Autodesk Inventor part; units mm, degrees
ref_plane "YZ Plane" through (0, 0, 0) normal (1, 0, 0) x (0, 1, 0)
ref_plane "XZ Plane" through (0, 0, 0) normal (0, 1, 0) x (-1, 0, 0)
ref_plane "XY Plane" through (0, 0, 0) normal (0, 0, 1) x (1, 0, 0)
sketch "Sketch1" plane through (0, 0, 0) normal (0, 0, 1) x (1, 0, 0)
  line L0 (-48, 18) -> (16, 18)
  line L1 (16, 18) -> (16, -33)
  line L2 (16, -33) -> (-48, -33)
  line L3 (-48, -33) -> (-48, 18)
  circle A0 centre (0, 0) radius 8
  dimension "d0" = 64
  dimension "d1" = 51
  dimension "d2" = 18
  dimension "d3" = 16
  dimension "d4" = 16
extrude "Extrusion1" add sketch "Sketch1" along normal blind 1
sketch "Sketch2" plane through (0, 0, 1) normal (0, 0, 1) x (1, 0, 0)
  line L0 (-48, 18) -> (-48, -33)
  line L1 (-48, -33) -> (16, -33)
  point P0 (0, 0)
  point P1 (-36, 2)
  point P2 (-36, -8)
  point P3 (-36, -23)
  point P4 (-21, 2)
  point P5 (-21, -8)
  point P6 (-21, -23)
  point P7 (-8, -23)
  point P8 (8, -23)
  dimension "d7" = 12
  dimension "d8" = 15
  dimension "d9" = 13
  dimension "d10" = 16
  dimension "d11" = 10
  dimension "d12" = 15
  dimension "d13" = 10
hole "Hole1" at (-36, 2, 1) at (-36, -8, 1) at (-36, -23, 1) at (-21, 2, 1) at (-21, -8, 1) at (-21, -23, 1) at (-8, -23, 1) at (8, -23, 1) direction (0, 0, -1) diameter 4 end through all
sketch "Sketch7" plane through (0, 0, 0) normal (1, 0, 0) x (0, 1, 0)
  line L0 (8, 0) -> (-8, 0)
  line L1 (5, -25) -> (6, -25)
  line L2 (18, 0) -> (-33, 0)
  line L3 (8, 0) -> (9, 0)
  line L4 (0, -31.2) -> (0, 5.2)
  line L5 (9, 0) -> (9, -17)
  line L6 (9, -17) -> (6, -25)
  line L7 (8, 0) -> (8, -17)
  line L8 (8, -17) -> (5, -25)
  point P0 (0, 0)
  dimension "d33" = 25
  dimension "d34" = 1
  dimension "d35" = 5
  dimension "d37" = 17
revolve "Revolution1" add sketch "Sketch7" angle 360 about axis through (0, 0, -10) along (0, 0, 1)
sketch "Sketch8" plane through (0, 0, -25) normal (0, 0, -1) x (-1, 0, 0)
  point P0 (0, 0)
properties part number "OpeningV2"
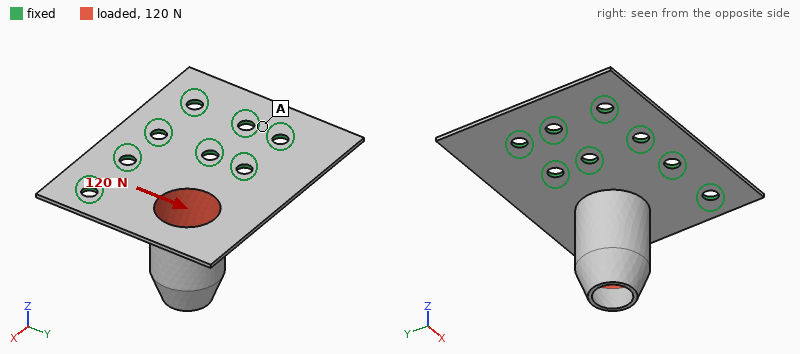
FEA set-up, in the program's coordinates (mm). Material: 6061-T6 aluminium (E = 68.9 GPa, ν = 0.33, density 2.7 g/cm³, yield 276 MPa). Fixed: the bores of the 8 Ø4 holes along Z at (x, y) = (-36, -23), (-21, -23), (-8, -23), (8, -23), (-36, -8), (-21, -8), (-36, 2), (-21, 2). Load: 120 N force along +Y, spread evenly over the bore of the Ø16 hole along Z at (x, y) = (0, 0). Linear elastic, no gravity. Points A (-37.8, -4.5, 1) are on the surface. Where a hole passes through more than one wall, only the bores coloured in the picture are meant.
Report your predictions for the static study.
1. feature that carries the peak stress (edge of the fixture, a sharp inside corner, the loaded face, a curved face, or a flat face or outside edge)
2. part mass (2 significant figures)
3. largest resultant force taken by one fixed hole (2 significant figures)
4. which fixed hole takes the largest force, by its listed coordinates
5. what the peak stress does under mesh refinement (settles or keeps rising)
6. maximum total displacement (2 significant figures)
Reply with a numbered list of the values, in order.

1. edge of the fixture
2. 11 g
3. 66 N
4. (8, -23)
5. keeps rising
6. 0.57 mm
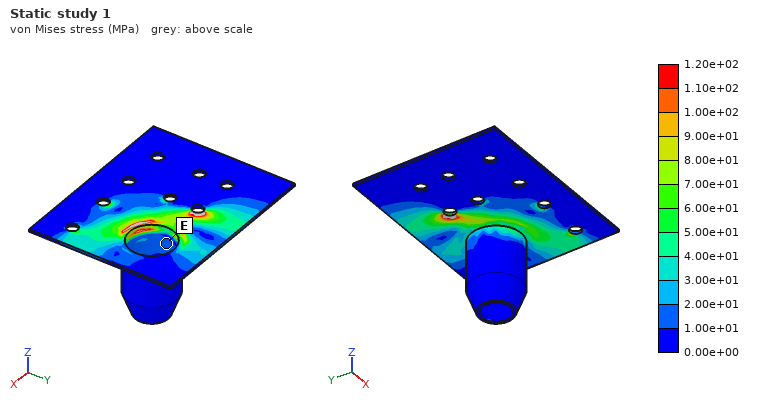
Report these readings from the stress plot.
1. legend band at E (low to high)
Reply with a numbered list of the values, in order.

1. 1.00e+01 to 2.00e+01 MPa
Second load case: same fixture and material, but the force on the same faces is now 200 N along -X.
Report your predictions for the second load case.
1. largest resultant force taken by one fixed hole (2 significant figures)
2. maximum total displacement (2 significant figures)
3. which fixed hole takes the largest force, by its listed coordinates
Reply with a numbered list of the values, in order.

1. 97 N
2. 0.92 mm
3. (-21, 2)
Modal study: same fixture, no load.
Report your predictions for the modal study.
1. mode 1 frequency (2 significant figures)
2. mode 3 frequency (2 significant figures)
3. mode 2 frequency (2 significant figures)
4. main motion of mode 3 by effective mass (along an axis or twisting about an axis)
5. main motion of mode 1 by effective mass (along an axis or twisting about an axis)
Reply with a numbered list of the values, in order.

1. 820 Hz
2. 3300 Hz
3. 2100 Hz
4. along Z
5. along Z
